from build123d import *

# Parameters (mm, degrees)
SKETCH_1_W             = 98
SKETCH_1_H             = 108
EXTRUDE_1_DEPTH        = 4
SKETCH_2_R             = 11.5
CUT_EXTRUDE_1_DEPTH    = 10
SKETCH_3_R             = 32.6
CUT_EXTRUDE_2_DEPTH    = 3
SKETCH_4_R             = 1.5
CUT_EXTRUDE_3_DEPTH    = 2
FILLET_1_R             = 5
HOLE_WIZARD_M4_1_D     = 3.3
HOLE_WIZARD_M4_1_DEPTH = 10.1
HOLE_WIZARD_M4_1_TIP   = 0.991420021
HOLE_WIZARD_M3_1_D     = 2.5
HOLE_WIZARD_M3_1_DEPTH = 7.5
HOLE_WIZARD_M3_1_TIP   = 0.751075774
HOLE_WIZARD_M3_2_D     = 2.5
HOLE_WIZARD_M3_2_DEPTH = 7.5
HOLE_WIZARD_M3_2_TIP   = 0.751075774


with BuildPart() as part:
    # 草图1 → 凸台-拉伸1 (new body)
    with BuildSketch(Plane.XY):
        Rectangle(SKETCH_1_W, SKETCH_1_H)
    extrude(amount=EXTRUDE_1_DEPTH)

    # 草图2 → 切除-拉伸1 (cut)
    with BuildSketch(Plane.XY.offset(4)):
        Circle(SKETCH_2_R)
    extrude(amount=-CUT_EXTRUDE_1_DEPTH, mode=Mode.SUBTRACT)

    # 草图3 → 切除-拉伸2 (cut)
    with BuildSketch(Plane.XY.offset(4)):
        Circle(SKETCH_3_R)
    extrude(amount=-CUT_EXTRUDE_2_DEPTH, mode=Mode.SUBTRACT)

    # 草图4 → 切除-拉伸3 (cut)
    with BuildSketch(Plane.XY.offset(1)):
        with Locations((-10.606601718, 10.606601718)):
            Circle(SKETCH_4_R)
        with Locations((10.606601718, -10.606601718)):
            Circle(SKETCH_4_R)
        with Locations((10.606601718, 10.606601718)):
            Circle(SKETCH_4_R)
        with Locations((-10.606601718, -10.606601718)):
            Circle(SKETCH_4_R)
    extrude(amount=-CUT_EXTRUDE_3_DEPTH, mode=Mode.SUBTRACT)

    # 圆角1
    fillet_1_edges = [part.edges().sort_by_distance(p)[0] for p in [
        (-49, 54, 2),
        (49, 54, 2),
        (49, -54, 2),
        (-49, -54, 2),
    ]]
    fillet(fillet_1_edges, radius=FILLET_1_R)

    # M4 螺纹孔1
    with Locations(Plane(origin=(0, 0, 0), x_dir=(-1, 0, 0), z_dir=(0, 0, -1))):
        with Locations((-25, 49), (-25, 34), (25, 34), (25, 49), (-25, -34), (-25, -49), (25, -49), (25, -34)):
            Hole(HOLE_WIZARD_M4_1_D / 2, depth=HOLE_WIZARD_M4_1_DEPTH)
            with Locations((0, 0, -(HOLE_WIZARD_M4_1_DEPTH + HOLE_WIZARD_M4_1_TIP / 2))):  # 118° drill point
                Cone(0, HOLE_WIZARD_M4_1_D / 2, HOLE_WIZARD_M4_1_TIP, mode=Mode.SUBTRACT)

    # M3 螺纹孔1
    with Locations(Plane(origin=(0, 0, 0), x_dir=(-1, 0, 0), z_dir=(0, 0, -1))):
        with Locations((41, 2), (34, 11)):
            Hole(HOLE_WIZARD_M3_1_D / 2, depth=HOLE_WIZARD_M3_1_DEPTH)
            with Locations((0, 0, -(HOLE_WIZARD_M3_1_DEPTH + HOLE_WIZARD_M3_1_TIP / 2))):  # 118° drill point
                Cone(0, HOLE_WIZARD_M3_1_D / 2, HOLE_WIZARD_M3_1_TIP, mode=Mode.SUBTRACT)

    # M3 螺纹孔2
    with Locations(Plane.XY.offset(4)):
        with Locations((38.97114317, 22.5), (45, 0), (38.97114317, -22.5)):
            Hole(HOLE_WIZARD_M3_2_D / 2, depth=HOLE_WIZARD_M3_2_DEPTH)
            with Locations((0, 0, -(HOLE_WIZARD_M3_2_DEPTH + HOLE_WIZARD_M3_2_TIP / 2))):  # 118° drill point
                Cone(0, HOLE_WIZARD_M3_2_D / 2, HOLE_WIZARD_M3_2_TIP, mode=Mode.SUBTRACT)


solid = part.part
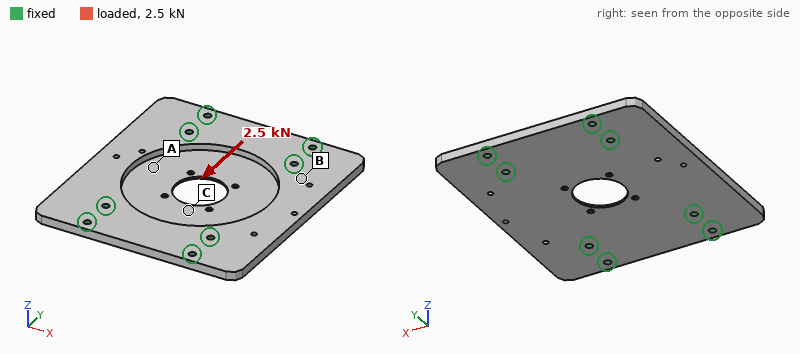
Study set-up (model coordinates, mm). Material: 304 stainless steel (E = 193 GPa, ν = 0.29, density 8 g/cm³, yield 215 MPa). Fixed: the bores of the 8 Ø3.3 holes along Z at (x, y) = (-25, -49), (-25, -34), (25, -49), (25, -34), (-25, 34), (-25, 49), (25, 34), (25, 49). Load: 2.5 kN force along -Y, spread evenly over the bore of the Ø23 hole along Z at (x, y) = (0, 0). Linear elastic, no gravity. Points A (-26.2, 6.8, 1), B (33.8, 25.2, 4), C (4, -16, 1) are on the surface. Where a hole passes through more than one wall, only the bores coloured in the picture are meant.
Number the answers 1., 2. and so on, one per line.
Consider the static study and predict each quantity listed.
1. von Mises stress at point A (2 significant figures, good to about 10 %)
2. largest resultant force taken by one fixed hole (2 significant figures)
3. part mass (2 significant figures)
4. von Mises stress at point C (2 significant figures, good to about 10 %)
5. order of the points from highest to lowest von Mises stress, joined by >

1. 11 MPa
2. 440 N
3. 250 g
4. 32 MPa
5. C > A > B
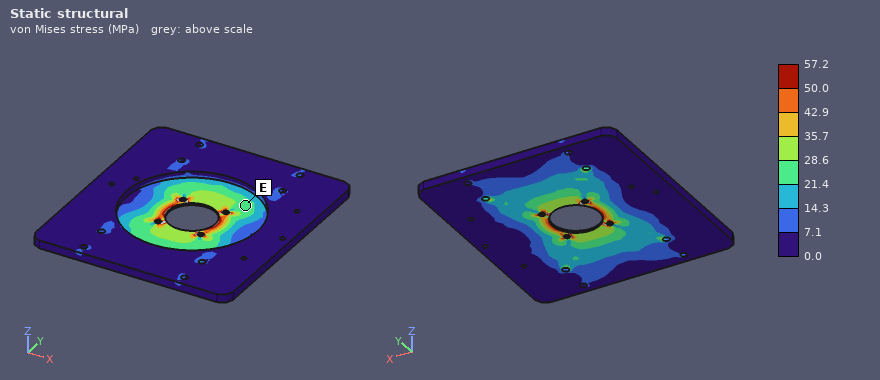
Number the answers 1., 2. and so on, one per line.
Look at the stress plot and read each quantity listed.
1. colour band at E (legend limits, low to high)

1. 21.4 to 28.6 MPa
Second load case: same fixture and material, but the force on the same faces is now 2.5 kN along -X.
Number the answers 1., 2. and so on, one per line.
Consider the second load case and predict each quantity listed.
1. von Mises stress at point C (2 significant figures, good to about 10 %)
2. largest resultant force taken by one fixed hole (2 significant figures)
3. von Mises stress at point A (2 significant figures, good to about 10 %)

1. 36 MPa
2. 600 N
3. 22 MPa
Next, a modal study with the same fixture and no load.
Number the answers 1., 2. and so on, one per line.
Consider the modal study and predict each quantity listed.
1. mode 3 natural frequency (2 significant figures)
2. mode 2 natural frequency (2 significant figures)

1. 3100 Hz
2. 3100 Hz
